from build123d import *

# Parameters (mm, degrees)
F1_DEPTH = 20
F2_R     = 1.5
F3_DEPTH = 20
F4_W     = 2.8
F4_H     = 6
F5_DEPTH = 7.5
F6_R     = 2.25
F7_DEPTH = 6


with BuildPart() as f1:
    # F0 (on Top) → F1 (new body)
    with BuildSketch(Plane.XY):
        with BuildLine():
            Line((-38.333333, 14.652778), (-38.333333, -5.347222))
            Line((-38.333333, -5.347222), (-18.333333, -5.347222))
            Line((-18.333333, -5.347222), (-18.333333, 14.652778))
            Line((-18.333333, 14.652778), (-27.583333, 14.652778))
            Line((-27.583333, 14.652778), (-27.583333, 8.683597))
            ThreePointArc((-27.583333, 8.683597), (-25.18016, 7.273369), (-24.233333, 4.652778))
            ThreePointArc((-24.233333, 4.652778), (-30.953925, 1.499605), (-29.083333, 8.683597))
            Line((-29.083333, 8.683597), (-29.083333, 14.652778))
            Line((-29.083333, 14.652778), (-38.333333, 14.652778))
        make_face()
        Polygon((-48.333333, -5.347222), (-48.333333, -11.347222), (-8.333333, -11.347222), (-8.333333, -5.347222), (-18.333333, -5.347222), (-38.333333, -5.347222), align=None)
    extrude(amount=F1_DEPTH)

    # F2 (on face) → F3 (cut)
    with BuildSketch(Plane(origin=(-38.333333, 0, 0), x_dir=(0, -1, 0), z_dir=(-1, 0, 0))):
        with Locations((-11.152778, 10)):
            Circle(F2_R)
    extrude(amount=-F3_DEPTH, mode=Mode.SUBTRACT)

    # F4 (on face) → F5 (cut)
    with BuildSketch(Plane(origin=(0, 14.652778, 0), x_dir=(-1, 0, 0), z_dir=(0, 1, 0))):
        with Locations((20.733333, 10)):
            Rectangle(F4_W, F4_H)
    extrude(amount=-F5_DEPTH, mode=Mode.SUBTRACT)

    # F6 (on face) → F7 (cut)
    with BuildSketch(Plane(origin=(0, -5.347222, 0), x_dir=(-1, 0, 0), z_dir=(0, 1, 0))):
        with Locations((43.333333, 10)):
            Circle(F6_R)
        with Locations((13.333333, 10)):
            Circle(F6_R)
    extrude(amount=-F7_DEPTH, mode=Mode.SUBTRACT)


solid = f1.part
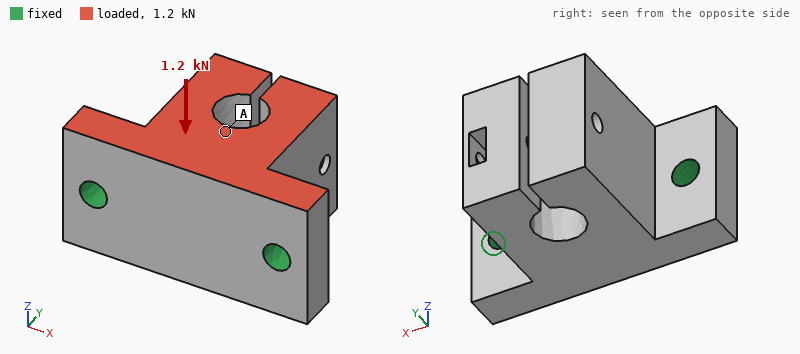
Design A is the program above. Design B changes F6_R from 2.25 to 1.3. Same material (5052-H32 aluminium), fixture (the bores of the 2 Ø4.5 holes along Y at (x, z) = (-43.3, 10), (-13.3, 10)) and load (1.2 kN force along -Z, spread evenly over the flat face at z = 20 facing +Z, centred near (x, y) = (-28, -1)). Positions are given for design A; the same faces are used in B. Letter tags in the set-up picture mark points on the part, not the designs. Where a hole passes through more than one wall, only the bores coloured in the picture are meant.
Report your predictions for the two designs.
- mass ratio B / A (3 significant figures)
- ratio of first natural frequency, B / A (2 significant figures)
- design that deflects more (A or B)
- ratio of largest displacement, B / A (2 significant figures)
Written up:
1.01
0.83
B
1.4
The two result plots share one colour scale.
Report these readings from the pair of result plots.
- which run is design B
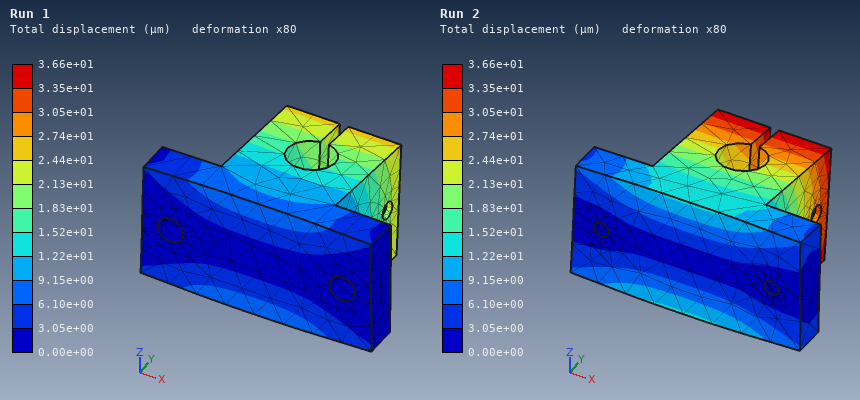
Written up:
Run 2
